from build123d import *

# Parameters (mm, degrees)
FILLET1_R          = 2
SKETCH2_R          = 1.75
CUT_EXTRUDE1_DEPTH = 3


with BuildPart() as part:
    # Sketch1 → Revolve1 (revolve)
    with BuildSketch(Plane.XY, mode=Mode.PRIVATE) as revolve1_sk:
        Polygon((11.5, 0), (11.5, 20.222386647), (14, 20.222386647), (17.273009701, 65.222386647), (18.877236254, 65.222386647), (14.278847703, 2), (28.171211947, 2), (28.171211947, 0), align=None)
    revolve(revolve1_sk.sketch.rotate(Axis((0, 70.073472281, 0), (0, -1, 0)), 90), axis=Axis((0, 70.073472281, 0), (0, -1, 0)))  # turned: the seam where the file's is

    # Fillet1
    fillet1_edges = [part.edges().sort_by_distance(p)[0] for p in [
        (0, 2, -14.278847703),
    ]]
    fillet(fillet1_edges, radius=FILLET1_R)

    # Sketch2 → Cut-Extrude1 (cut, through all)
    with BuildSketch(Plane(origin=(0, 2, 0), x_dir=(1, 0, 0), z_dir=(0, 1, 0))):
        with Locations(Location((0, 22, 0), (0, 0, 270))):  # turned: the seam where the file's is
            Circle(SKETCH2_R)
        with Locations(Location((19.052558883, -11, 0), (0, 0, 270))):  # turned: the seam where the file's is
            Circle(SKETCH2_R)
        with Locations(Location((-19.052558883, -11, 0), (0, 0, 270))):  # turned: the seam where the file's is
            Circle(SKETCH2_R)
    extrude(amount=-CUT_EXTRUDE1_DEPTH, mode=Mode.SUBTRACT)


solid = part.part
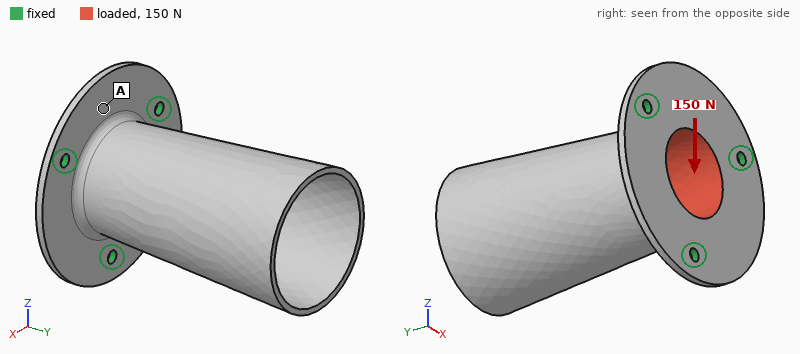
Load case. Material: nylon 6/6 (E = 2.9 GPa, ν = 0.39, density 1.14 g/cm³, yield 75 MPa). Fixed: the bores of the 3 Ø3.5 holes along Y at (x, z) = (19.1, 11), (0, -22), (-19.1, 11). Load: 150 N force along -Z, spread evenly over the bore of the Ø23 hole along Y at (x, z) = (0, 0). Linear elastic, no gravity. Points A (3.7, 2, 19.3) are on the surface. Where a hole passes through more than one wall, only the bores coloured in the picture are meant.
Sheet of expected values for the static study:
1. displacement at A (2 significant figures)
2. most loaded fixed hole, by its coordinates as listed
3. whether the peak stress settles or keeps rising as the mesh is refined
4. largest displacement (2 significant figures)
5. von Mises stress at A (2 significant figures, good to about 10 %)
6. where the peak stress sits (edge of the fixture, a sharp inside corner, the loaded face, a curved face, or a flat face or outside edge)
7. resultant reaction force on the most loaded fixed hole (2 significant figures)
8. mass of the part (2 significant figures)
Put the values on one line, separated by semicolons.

0.083 mm; (0, -22); keeps rising; 0.30 mm; 1.3 MPa; edge of the fixture; 70 N; 19 g
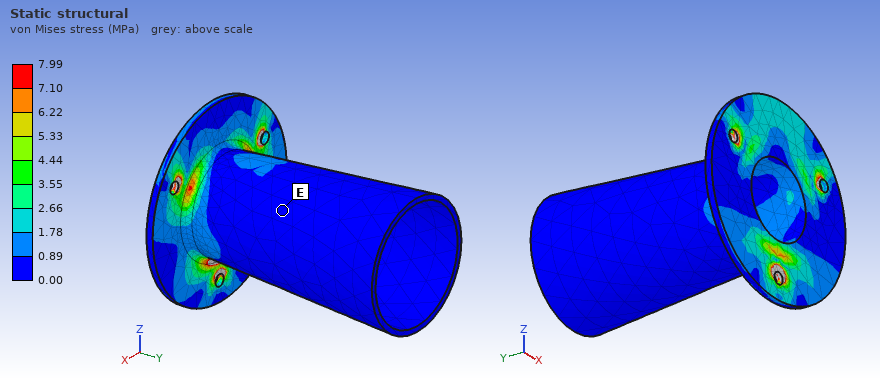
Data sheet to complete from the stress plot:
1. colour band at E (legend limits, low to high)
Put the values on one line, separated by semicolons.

0.00 to 0.89 MPa
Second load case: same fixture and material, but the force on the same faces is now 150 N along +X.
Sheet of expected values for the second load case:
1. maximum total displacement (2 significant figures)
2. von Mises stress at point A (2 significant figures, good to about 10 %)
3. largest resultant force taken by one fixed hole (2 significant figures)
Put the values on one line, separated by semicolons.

0.29 mm; 1.3 MPa; 65 N
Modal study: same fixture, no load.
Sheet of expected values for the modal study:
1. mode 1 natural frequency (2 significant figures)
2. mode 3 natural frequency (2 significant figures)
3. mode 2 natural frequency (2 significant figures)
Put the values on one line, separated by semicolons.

600 Hz; 1300 Hz; 600 Hz
